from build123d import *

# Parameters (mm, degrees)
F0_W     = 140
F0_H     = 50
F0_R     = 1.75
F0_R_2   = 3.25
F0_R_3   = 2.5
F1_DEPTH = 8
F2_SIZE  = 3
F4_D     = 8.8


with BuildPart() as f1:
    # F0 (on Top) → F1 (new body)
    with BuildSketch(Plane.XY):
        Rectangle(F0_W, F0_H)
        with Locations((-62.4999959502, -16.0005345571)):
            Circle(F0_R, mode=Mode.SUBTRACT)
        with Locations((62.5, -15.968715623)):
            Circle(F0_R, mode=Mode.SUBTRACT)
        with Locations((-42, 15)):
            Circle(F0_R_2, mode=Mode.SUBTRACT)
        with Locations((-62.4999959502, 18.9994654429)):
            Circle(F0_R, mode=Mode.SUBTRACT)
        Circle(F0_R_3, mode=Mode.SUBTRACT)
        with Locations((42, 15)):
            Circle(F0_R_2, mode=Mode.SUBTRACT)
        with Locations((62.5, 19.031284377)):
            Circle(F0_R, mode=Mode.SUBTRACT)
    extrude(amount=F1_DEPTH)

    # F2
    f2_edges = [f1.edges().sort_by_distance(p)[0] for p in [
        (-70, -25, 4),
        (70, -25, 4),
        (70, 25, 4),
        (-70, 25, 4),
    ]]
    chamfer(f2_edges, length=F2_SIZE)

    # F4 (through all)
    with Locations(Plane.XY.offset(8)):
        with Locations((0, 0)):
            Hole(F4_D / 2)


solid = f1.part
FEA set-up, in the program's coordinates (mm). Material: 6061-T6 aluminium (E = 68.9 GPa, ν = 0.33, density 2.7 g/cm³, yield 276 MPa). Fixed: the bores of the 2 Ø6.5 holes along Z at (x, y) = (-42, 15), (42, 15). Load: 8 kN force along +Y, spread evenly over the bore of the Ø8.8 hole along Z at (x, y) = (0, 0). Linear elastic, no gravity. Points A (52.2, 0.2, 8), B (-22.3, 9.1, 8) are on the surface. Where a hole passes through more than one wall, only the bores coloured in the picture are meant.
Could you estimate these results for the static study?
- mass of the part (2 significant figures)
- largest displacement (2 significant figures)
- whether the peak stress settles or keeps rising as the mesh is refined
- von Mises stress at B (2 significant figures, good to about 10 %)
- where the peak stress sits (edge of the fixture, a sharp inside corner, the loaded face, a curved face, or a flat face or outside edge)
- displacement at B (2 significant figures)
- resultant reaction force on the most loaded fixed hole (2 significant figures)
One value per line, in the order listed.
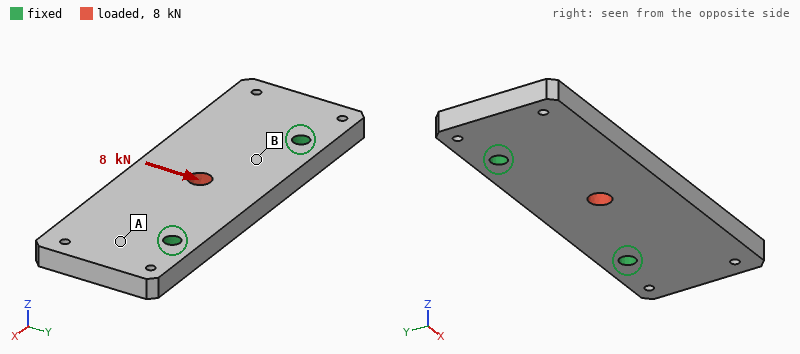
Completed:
150 g
33 µm
keeps rising
24 MPa
edge of the fixture
17 µm
4.7 kN
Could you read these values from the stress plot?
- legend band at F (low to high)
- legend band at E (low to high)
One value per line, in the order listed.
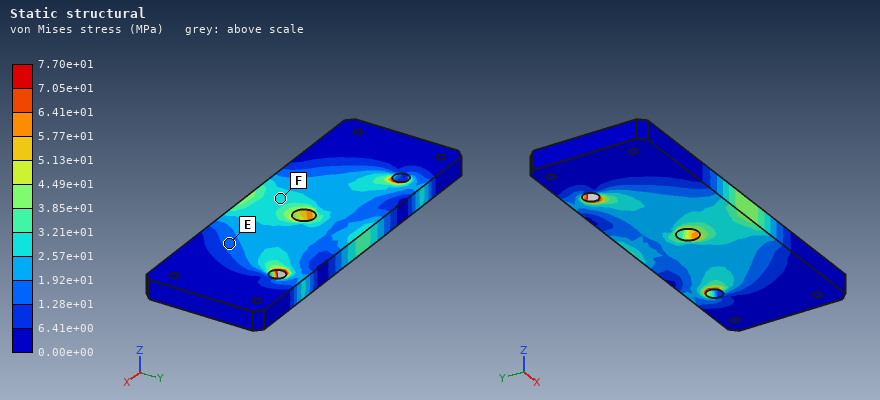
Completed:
2.57e+01 to 3.21e+01 MPa
1.28e+01 to 1.92e+01 MPa
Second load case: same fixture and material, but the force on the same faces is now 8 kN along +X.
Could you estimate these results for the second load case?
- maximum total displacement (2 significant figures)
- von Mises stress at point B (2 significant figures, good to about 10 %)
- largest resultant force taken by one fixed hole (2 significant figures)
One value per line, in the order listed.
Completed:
17 µm
21 MPa
4.2 kN
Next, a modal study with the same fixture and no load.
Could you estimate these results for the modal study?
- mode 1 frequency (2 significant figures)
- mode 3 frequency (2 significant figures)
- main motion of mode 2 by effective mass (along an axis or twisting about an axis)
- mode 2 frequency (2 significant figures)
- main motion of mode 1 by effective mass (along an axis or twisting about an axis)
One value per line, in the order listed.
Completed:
2800 Hz
4300 Hz
twisting about Y
3900 Hz
along Z
